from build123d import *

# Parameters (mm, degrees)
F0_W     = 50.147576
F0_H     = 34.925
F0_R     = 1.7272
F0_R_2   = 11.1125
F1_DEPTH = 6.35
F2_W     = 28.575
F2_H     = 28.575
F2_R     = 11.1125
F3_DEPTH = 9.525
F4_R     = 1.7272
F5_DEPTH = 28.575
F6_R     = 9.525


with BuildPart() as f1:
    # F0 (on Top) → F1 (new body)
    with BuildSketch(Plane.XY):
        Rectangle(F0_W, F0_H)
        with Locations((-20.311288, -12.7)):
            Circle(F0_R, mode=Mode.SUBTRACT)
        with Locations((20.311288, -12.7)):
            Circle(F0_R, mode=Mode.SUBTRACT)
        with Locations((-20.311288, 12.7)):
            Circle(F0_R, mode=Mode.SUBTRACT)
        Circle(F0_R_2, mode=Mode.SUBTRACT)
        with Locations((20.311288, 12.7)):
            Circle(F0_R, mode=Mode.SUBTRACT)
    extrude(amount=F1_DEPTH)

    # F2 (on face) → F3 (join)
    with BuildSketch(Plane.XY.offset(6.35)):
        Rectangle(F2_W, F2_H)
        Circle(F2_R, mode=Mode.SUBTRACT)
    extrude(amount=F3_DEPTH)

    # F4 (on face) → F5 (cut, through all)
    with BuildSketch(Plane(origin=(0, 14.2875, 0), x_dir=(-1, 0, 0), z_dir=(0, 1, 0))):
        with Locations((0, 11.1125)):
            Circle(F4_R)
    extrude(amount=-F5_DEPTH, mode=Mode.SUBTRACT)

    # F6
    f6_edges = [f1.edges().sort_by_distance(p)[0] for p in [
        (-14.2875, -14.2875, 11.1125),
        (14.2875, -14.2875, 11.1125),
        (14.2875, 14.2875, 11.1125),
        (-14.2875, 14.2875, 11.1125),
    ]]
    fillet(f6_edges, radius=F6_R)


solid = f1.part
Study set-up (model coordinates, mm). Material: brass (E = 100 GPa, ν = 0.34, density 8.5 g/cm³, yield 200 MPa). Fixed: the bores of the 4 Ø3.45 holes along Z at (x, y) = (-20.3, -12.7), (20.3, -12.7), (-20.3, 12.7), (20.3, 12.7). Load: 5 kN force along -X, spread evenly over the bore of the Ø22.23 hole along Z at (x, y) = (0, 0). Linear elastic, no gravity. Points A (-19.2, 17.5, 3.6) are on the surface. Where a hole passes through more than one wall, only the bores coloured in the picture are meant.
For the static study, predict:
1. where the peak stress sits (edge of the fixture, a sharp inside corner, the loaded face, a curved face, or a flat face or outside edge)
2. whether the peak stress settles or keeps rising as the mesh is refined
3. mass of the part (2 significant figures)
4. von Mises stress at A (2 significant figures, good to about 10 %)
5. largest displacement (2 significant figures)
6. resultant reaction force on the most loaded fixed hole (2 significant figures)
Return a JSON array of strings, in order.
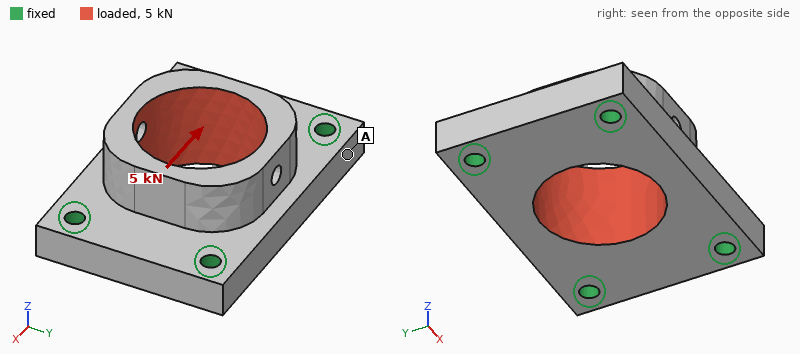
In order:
["edge of the fixture", "keeps rising", "99 g", "7.8 MPa", "8.9 µm", "1.3 kN"]
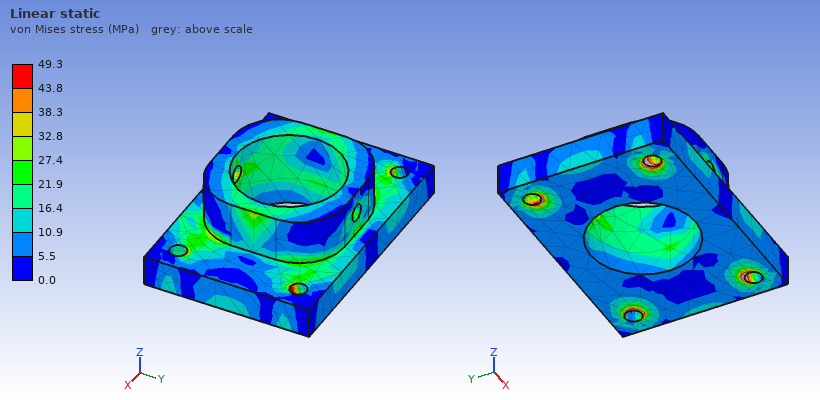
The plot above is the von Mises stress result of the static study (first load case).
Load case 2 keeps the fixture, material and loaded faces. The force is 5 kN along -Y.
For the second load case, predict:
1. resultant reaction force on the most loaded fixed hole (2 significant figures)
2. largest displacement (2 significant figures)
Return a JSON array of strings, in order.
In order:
["1.5 kN", "16 µm"]
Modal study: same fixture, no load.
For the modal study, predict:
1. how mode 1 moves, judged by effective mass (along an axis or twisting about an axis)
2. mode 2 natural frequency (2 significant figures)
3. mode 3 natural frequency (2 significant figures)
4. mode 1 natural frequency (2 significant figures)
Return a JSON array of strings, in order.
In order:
["along Z", "13 kHz", "18 kHz", "12 kHz"]
